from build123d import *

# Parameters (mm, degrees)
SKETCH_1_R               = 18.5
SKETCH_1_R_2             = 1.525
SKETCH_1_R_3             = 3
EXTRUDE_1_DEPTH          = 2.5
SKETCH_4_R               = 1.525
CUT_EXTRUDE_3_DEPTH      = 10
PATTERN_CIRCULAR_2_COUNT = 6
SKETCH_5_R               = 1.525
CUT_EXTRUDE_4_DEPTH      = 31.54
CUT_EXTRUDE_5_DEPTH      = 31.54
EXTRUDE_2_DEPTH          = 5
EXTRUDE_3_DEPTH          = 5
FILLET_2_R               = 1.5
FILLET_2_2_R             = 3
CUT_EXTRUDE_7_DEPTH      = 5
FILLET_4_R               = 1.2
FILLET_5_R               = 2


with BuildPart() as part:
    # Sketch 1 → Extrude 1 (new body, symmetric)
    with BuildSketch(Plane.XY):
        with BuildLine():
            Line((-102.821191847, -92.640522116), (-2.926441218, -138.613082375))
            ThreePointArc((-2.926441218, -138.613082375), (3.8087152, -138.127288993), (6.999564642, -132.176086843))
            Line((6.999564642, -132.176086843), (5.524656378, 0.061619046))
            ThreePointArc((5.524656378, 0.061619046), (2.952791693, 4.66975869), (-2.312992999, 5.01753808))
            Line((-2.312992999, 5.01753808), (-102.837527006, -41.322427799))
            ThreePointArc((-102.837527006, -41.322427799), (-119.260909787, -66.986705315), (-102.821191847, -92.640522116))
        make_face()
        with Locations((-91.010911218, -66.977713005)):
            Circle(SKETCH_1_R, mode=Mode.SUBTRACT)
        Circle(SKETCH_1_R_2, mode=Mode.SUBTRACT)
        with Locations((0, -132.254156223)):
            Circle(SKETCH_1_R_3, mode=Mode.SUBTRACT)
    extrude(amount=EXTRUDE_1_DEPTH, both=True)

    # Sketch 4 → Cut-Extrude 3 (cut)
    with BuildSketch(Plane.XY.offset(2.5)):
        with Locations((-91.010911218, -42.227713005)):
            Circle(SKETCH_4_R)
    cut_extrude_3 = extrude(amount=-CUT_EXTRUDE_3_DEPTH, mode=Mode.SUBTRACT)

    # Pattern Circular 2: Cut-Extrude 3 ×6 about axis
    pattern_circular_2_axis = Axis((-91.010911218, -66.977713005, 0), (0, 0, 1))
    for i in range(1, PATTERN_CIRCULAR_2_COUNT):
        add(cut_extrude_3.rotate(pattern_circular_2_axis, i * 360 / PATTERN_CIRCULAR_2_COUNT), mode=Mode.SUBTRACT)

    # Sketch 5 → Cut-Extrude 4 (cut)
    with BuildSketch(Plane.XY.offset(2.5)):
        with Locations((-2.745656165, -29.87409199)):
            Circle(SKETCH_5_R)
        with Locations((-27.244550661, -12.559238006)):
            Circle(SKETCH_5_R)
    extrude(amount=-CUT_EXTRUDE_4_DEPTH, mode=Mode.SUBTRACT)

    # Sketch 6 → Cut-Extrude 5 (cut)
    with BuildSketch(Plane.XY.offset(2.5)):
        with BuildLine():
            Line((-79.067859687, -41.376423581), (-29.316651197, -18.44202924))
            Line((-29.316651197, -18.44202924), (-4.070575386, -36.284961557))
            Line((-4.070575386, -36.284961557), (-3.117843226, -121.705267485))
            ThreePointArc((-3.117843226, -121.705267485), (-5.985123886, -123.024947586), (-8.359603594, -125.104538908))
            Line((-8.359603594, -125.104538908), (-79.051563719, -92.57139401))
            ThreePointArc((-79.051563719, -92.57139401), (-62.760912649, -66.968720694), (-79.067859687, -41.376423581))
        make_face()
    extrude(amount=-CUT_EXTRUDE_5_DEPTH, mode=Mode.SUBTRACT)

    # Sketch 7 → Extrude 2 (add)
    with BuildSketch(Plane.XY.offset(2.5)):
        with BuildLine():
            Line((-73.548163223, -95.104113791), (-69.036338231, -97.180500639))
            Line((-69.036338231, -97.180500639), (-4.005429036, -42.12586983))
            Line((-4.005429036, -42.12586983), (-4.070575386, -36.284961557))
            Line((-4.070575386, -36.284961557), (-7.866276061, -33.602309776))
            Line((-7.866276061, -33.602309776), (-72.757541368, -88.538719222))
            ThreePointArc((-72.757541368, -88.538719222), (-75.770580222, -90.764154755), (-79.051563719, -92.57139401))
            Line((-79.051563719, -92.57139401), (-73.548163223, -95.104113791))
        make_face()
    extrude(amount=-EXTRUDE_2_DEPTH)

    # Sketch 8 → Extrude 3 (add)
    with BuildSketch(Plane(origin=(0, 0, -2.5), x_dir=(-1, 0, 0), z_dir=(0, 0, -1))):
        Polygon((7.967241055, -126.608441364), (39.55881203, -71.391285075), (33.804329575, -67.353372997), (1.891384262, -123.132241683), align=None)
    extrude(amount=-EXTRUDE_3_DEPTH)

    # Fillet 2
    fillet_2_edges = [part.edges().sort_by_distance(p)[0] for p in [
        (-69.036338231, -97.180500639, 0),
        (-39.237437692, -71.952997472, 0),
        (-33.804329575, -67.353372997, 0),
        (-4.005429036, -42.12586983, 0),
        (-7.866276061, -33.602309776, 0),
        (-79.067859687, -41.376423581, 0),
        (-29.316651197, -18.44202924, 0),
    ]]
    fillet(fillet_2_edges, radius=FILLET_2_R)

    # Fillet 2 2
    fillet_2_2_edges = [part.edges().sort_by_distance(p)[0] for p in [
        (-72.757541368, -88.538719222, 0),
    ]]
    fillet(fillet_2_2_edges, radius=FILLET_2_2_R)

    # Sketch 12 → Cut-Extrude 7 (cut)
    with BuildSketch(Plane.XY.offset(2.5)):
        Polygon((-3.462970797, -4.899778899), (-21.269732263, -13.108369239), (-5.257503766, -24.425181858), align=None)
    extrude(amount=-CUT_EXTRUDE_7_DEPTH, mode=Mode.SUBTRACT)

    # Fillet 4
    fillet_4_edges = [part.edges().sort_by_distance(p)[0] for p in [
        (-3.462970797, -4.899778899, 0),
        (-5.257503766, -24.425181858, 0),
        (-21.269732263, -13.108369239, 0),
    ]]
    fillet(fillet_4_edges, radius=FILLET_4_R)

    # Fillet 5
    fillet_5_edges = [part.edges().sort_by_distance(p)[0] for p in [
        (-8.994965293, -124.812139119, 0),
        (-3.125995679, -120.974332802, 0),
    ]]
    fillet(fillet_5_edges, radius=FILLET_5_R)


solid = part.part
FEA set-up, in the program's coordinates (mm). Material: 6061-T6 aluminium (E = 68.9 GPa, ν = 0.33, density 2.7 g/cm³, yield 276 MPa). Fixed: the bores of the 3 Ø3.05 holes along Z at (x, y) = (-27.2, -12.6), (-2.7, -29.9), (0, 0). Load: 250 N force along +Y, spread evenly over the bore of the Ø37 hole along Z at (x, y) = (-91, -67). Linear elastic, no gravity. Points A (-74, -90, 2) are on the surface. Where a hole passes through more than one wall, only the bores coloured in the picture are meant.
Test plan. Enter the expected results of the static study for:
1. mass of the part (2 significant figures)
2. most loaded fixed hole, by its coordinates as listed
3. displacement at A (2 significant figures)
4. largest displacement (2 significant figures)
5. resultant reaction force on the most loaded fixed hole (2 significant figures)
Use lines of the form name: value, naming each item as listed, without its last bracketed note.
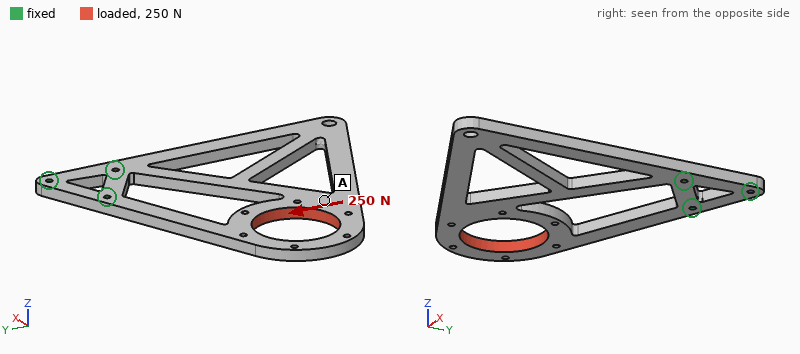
mass of the part: 83 g
most loaded fixed hole, by its coordinates as listed: (-27.2, -12.6)
displacement at A: 0.22 mm
largest displacement: 0.27 mm
resultant reaction force on the most loaded fixed hole: 440 N
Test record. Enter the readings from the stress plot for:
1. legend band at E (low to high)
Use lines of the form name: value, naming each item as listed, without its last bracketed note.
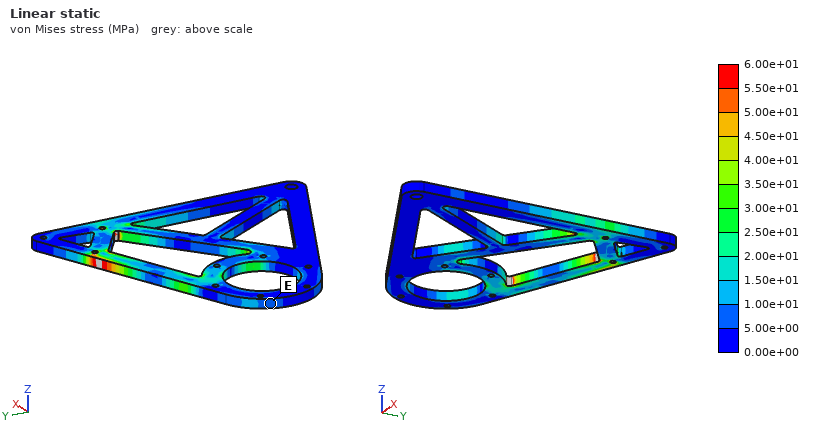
legend band at E: 5.00e+00 to 1.00e+01 MPa
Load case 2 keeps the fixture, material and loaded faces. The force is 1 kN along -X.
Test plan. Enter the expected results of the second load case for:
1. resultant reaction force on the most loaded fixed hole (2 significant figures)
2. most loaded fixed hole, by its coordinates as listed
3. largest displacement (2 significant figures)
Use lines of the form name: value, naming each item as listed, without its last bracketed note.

resultant reaction force on the most loaded fixed hole: 1.3 kN
most loaded fixed hole, by its coordinates as listed: (-2.7, -29.9)
largest displacement: 0.64 mm
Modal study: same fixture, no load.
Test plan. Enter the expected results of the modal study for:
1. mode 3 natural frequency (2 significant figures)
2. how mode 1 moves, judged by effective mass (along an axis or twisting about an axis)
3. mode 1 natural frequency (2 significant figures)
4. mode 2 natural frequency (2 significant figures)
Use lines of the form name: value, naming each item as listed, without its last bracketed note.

mode 3 natural frequency: 710 Hz
how mode 1 moves, judged by effective mass: along Z
mode 1 natural frequency: 220 Hz
mode 2 natural frequency: 380 Hz
